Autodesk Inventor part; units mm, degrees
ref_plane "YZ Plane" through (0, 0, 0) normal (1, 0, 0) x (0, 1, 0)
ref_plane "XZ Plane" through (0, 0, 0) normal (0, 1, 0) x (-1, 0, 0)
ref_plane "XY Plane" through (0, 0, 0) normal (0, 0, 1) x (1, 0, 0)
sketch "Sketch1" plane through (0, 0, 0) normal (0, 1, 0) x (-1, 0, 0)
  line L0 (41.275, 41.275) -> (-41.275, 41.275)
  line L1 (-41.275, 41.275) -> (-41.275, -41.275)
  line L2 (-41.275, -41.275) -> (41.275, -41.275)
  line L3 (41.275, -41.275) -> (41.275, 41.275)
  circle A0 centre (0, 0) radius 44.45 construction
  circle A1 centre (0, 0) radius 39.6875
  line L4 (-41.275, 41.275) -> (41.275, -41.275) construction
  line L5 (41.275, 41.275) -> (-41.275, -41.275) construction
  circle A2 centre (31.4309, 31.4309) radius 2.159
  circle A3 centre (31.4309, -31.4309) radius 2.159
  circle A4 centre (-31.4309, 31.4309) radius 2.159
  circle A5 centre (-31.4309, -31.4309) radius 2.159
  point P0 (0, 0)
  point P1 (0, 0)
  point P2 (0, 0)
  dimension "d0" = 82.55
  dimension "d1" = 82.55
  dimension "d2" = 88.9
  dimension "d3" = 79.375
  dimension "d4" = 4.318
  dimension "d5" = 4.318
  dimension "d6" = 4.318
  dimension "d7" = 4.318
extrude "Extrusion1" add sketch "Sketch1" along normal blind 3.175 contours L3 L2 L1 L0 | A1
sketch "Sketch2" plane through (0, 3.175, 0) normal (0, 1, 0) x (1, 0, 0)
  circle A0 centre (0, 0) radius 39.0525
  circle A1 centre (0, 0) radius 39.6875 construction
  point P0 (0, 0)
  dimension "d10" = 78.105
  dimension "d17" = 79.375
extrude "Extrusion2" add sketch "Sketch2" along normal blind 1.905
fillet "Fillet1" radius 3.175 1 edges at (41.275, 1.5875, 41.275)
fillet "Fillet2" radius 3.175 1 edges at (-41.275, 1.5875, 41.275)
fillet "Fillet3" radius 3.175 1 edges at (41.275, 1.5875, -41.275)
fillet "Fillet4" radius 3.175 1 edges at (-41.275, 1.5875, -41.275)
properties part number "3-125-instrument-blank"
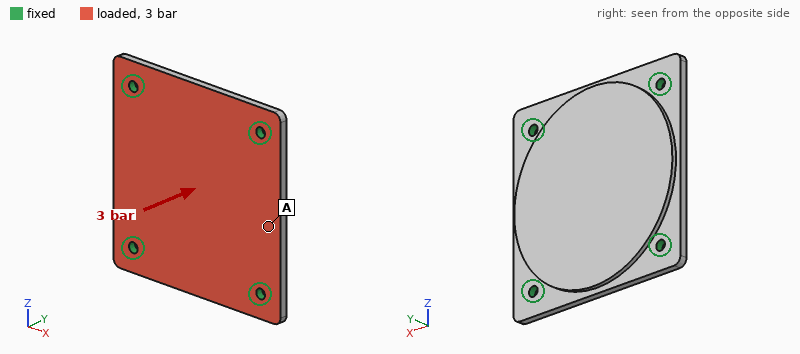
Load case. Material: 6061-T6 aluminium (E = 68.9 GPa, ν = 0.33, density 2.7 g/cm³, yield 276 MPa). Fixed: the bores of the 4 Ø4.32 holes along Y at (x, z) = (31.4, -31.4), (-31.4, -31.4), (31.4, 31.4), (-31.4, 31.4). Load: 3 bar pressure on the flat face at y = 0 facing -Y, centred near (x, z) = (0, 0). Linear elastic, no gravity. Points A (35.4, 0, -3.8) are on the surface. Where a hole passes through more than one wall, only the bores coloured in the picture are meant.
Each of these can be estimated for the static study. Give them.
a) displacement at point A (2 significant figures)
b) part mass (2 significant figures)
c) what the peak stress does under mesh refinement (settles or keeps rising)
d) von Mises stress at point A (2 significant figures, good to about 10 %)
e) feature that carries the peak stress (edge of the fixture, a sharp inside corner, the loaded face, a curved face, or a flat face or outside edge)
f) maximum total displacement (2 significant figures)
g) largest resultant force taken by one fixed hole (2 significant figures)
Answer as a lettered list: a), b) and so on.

a) 35 µm
b) 82 g
c) keeps rising
d) 17 MPa
e) edge of the fixture
f) 62 µm
g) 710 N
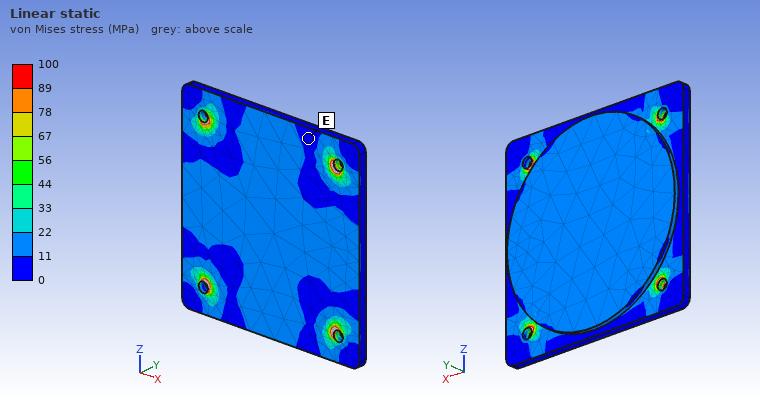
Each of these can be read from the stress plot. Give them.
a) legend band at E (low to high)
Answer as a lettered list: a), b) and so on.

a) 0 to 11 MPa
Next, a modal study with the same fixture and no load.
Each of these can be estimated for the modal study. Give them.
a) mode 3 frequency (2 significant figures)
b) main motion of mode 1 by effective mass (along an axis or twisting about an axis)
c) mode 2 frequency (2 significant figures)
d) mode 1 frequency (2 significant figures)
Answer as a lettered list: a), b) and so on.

a) 5700 Hz
b) along Y
c) 5700 Hz
d) 3600 Hz
